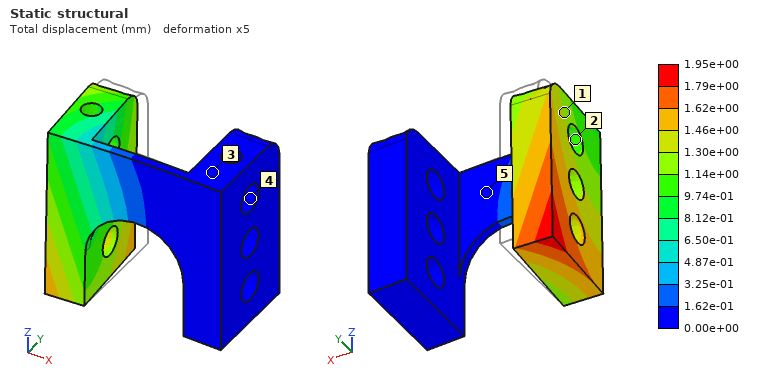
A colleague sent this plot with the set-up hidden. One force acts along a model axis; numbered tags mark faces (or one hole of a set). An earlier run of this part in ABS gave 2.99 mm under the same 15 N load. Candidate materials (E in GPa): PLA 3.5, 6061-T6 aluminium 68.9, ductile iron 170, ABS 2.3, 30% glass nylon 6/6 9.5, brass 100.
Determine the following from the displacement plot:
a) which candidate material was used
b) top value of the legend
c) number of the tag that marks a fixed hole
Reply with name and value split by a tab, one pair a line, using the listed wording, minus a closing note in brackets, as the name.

which candidate material was used	PLA
top value of the legend	1.95e+00 mm
number of the tag that marks a fixed hole	4
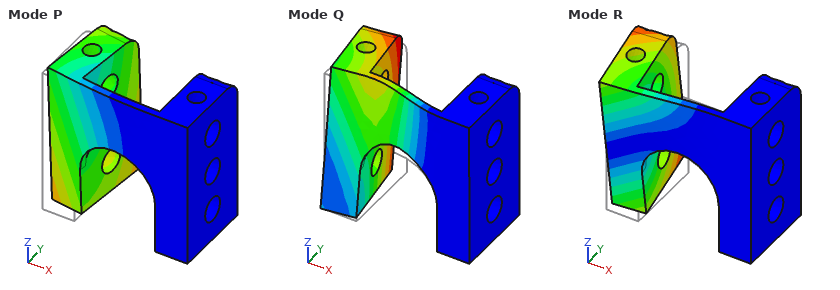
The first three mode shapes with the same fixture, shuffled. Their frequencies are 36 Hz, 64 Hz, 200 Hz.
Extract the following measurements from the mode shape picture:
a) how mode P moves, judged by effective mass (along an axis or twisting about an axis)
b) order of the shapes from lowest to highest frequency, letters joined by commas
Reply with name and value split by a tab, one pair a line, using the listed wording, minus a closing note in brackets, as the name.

how mode P moves, judged by effective mass	along Y
order of the shapes from lowest to highest frequency, letters joined by commas	P, R, Q
